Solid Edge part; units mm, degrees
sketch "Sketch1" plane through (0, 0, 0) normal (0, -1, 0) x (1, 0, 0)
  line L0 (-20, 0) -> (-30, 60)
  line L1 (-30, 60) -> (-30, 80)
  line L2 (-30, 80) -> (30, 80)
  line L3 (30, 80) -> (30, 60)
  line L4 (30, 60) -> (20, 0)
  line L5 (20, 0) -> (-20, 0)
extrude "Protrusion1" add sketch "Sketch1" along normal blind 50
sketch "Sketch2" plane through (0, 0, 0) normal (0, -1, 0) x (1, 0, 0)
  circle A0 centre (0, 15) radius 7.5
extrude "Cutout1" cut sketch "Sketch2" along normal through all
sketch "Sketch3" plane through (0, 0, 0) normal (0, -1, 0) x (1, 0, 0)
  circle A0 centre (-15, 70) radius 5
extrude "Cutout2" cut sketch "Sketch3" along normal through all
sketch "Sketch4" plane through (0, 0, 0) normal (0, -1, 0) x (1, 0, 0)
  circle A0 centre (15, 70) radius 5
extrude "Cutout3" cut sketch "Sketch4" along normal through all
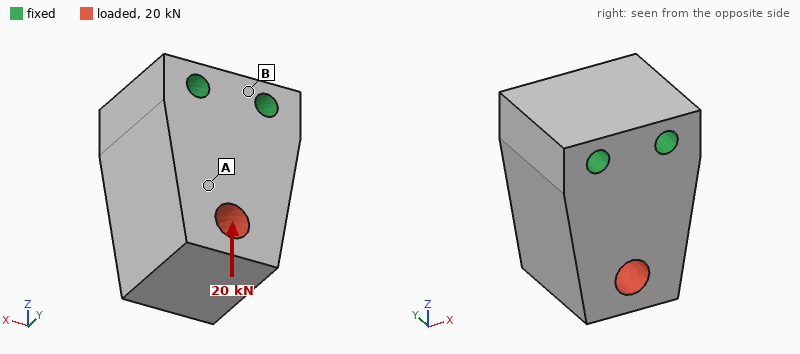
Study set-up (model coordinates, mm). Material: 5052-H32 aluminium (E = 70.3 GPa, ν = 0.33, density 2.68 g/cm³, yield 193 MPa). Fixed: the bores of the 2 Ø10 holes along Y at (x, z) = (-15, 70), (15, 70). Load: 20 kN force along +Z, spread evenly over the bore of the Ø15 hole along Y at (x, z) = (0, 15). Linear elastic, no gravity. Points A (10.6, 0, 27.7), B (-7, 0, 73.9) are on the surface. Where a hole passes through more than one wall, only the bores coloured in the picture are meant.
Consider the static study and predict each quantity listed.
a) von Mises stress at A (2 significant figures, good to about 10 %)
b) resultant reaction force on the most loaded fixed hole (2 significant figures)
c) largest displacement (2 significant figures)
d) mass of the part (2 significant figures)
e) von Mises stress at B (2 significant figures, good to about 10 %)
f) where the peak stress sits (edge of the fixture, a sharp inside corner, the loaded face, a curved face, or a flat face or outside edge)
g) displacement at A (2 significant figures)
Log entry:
11 MPa
10 kN
11 µm
520 g
5.0 MPa
the loaded face
4.9 µm
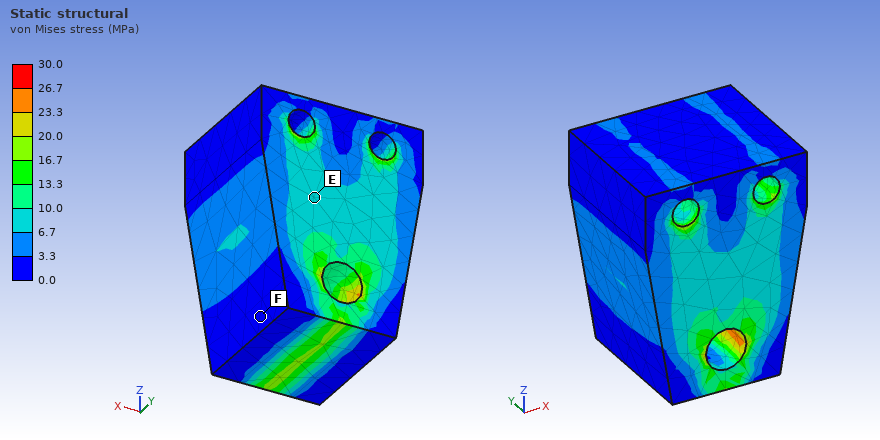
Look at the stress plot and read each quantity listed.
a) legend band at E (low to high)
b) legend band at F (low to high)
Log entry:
6.7 to 10.0 MPa
0.0 to 3.3 MPa
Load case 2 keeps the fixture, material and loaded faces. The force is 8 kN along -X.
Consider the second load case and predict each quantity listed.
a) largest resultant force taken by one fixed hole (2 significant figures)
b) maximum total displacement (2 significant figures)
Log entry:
12 kN
23 µm
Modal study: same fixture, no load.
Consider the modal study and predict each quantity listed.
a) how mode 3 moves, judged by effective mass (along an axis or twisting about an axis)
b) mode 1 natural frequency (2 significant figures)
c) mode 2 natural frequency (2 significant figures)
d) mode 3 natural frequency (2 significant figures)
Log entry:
twisting about Z
7500 Hz
7700 Hz
13 kHz
